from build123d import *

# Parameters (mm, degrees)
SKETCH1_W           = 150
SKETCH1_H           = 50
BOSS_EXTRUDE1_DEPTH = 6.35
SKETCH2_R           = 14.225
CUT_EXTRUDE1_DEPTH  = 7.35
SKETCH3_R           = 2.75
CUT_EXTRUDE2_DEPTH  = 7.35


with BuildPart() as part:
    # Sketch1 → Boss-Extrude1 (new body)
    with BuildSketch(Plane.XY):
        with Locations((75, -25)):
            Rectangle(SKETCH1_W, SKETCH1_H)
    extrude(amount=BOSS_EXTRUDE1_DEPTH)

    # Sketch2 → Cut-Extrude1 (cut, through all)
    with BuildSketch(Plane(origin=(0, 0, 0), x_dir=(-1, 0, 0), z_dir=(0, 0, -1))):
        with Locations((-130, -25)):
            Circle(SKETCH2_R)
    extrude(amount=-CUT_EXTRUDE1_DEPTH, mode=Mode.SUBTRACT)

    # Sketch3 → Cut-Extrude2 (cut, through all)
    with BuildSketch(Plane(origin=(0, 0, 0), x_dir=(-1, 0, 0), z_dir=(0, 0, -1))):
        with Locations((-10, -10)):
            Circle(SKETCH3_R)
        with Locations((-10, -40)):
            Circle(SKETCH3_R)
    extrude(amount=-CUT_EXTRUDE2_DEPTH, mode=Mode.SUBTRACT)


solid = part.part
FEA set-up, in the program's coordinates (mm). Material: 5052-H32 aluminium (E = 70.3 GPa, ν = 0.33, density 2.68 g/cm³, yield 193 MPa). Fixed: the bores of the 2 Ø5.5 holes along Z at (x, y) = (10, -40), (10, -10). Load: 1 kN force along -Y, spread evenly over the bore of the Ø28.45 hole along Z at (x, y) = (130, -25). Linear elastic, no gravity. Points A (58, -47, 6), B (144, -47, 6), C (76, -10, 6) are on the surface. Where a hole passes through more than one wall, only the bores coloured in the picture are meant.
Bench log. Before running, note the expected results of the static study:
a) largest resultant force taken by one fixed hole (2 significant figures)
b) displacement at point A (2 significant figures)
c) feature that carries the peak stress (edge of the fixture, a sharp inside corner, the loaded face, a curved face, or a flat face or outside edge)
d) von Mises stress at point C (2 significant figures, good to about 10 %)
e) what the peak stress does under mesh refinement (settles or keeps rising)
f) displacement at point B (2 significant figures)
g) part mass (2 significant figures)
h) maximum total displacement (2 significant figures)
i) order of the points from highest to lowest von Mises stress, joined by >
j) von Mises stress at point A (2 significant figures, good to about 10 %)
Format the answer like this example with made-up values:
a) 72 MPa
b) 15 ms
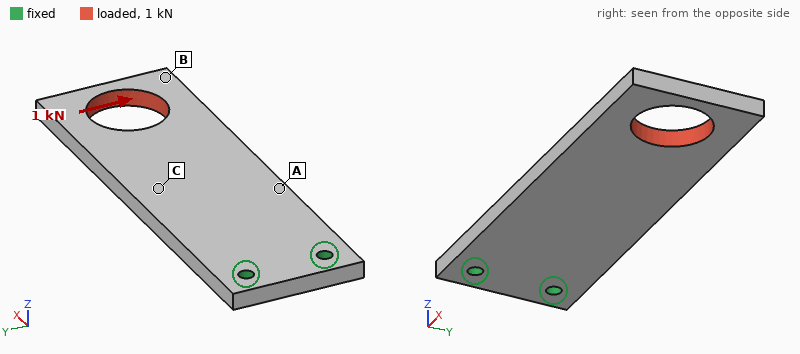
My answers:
a) 3.7 kN
b) 0.045 mm
c) edge of the fixture
d) 13 MPa
e) keeps rising
f) 0.19 mm
g) 120 g
h) 0.21 mm
i) A > C > B
j) 24 MPa
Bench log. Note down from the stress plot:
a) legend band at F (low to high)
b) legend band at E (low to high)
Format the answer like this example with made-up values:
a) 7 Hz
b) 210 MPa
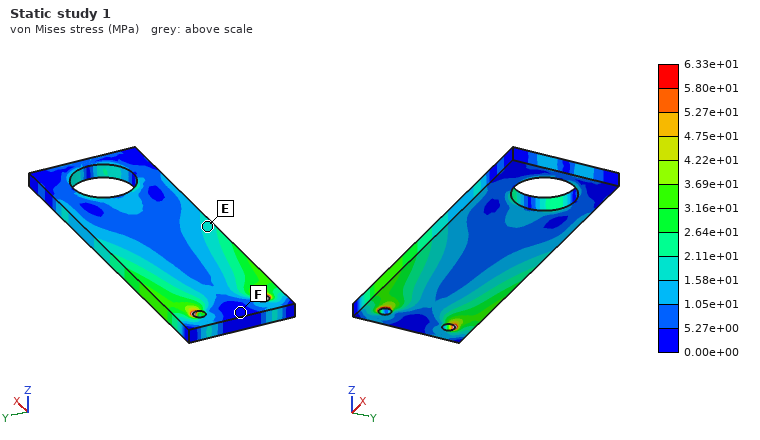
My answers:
a) 0.00e+00 to 5.27e+00 MPa
b) 1.58e+01 to 2.11e+01 MPa
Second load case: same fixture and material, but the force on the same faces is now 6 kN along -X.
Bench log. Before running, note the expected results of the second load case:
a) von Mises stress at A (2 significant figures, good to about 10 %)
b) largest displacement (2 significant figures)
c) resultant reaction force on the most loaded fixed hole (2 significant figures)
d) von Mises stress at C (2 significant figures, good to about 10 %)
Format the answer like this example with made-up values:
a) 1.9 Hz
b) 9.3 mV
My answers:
a) 19 MPa
b) 66 µm
c) 3.0 kN
d) 19 MPa
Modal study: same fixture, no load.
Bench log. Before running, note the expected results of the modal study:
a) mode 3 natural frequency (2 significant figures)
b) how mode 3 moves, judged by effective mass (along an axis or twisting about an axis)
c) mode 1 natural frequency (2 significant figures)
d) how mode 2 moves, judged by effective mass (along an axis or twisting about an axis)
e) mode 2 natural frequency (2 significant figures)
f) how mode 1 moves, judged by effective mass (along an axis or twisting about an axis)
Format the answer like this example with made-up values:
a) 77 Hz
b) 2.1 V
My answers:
a) 1700 Hz
b) along Z
c) 310 Hz
d) twisting about X
e) 1500 Hz
f) along Z
